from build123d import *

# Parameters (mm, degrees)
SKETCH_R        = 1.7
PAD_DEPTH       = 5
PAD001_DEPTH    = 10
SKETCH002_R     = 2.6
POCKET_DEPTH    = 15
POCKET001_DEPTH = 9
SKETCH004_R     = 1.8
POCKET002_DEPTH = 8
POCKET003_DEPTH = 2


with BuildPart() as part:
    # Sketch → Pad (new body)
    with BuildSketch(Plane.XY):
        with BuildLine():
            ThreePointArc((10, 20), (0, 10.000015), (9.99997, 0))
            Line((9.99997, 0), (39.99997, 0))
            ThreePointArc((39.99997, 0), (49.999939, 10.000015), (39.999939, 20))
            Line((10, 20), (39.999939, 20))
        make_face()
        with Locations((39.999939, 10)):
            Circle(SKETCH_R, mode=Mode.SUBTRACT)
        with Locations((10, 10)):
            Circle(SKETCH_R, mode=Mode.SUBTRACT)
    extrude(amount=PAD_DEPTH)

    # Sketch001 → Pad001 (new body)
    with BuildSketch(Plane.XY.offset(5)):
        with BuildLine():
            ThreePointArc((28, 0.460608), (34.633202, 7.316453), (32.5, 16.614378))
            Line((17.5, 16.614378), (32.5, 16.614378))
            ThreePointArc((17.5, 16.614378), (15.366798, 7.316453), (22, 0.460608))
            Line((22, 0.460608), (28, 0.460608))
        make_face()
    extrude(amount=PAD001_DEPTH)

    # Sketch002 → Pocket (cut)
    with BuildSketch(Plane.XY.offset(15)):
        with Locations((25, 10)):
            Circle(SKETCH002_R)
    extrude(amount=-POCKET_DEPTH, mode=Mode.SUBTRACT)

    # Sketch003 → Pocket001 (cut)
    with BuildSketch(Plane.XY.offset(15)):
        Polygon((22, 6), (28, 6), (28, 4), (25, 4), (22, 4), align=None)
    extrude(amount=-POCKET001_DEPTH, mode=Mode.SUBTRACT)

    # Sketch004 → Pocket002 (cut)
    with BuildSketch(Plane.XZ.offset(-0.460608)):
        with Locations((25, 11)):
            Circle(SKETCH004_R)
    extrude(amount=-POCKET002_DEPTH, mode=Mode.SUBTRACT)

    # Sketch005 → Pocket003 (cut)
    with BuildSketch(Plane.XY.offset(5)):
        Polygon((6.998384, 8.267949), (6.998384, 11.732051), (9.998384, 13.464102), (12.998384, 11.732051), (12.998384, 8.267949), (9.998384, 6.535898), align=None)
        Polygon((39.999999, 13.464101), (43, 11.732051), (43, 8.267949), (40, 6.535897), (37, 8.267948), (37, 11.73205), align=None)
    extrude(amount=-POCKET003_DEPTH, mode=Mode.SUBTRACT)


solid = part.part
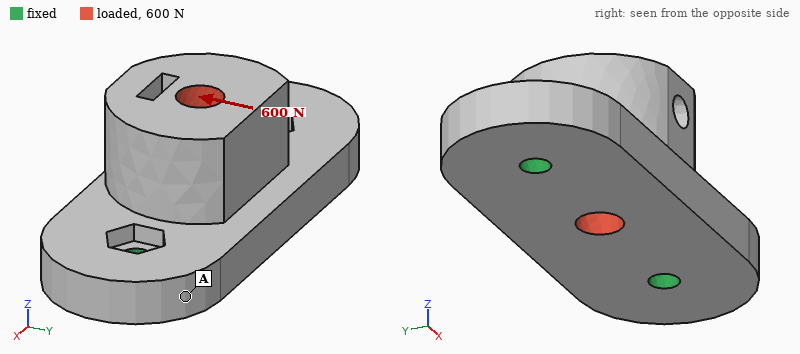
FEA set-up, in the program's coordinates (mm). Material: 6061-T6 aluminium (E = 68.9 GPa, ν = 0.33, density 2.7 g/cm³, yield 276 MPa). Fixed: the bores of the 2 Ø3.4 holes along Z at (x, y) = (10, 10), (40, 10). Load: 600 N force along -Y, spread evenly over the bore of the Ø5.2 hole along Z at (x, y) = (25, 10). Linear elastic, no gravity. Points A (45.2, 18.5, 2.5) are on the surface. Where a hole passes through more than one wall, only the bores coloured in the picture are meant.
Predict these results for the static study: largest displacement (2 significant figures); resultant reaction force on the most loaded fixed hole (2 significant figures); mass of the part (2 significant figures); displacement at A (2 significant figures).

23 µm
300 N
18 g
6.6 µm
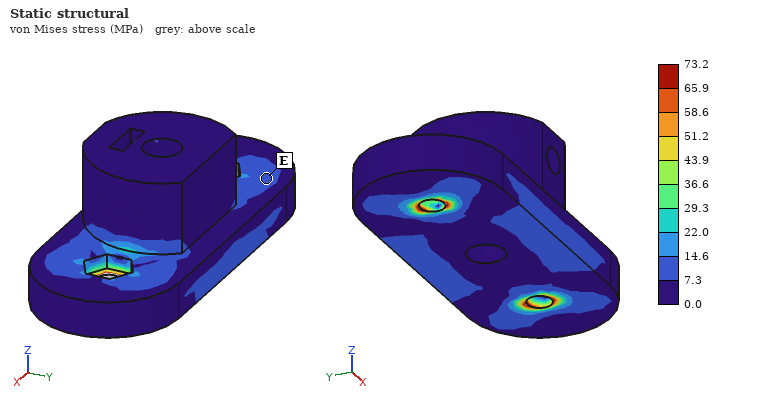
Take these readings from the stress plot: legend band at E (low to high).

7.3 to 14.6 MPa
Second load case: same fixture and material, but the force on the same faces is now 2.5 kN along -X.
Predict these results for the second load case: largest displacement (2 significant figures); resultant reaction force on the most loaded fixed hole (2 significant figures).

9.9 µm
1.4 kN
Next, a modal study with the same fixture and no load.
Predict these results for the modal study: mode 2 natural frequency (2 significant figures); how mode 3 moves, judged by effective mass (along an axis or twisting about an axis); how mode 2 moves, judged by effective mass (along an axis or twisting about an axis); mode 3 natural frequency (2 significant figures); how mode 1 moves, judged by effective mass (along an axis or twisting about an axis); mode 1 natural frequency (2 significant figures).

18 kHz
along X
along Z
27 kHz
along Y
8400 Hz
